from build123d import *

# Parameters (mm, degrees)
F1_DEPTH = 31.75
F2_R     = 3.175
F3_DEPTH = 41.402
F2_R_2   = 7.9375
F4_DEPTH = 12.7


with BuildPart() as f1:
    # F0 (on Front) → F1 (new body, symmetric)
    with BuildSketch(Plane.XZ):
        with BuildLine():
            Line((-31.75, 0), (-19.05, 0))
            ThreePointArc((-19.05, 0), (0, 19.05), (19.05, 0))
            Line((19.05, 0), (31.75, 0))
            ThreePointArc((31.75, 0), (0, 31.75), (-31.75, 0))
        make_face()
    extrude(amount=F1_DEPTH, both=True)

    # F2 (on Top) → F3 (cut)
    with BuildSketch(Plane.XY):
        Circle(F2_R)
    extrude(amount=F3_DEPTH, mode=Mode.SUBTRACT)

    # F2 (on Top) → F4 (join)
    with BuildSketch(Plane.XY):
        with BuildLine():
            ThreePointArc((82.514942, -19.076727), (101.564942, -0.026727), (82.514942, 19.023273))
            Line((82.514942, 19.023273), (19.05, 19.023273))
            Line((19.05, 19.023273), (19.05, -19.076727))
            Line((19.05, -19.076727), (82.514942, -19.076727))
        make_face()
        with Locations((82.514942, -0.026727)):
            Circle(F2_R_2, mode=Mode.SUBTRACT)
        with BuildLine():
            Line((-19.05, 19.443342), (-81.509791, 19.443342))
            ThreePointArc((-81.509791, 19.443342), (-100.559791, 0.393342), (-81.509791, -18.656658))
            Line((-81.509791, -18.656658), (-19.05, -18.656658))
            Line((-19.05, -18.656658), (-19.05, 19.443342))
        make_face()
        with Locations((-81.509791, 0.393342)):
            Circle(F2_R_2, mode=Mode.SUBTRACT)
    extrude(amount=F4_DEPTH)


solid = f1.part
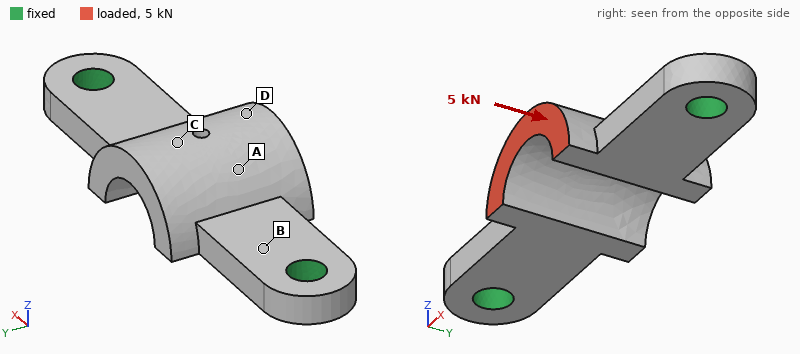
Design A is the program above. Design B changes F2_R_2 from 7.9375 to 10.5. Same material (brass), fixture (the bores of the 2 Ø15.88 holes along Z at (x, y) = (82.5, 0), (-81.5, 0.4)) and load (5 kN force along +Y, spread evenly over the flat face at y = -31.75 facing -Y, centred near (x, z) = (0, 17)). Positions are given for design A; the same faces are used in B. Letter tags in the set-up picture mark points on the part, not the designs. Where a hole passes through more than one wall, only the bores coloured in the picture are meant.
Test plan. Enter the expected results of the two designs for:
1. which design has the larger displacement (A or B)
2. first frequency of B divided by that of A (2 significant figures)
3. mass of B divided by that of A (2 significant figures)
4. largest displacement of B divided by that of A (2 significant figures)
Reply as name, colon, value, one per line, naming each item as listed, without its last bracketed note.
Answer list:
which design has the larger displacement: A
first frequency of B divided by that of A: 1.1
mass of B divided by that of A: 0.97
largest displacement of B divided by that of A: 0.89
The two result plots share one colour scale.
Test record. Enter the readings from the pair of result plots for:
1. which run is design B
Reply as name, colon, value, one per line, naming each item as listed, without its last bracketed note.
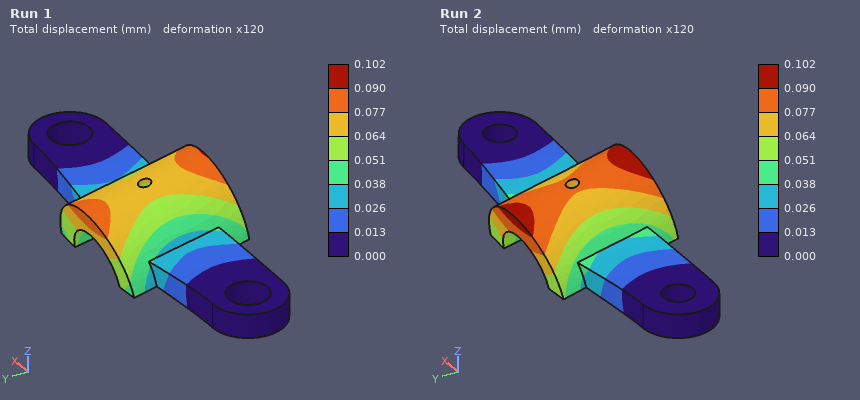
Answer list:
which run is design B: Run 1
